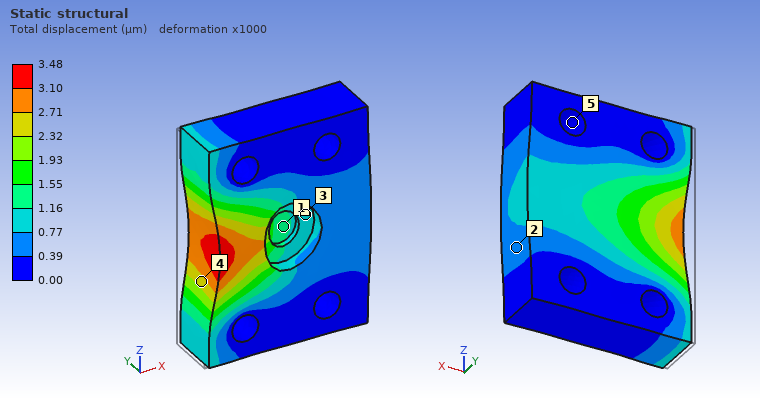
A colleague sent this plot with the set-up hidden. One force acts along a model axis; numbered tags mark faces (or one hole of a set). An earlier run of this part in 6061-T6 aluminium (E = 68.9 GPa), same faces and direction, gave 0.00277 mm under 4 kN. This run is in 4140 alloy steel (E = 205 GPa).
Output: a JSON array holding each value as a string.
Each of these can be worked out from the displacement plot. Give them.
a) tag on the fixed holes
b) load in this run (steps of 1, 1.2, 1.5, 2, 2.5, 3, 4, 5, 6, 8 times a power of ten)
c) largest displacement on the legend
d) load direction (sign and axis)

["5", "15 kN", "3.48 µm", "+X"]
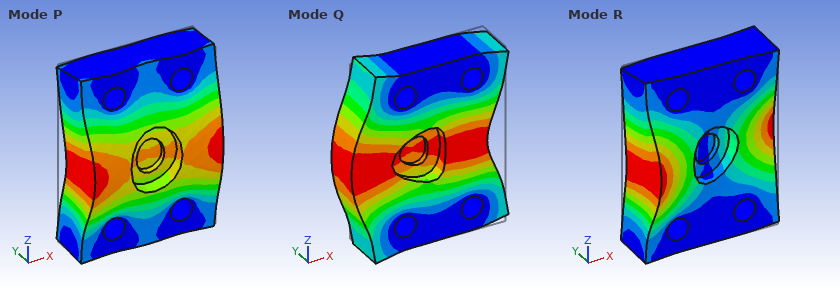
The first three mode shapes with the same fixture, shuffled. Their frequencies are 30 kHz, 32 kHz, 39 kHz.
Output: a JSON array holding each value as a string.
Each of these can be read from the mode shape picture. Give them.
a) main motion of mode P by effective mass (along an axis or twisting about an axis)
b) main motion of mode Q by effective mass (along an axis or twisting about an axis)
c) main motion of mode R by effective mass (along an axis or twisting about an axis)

["along Y", "along X", "twisting about Z"]
